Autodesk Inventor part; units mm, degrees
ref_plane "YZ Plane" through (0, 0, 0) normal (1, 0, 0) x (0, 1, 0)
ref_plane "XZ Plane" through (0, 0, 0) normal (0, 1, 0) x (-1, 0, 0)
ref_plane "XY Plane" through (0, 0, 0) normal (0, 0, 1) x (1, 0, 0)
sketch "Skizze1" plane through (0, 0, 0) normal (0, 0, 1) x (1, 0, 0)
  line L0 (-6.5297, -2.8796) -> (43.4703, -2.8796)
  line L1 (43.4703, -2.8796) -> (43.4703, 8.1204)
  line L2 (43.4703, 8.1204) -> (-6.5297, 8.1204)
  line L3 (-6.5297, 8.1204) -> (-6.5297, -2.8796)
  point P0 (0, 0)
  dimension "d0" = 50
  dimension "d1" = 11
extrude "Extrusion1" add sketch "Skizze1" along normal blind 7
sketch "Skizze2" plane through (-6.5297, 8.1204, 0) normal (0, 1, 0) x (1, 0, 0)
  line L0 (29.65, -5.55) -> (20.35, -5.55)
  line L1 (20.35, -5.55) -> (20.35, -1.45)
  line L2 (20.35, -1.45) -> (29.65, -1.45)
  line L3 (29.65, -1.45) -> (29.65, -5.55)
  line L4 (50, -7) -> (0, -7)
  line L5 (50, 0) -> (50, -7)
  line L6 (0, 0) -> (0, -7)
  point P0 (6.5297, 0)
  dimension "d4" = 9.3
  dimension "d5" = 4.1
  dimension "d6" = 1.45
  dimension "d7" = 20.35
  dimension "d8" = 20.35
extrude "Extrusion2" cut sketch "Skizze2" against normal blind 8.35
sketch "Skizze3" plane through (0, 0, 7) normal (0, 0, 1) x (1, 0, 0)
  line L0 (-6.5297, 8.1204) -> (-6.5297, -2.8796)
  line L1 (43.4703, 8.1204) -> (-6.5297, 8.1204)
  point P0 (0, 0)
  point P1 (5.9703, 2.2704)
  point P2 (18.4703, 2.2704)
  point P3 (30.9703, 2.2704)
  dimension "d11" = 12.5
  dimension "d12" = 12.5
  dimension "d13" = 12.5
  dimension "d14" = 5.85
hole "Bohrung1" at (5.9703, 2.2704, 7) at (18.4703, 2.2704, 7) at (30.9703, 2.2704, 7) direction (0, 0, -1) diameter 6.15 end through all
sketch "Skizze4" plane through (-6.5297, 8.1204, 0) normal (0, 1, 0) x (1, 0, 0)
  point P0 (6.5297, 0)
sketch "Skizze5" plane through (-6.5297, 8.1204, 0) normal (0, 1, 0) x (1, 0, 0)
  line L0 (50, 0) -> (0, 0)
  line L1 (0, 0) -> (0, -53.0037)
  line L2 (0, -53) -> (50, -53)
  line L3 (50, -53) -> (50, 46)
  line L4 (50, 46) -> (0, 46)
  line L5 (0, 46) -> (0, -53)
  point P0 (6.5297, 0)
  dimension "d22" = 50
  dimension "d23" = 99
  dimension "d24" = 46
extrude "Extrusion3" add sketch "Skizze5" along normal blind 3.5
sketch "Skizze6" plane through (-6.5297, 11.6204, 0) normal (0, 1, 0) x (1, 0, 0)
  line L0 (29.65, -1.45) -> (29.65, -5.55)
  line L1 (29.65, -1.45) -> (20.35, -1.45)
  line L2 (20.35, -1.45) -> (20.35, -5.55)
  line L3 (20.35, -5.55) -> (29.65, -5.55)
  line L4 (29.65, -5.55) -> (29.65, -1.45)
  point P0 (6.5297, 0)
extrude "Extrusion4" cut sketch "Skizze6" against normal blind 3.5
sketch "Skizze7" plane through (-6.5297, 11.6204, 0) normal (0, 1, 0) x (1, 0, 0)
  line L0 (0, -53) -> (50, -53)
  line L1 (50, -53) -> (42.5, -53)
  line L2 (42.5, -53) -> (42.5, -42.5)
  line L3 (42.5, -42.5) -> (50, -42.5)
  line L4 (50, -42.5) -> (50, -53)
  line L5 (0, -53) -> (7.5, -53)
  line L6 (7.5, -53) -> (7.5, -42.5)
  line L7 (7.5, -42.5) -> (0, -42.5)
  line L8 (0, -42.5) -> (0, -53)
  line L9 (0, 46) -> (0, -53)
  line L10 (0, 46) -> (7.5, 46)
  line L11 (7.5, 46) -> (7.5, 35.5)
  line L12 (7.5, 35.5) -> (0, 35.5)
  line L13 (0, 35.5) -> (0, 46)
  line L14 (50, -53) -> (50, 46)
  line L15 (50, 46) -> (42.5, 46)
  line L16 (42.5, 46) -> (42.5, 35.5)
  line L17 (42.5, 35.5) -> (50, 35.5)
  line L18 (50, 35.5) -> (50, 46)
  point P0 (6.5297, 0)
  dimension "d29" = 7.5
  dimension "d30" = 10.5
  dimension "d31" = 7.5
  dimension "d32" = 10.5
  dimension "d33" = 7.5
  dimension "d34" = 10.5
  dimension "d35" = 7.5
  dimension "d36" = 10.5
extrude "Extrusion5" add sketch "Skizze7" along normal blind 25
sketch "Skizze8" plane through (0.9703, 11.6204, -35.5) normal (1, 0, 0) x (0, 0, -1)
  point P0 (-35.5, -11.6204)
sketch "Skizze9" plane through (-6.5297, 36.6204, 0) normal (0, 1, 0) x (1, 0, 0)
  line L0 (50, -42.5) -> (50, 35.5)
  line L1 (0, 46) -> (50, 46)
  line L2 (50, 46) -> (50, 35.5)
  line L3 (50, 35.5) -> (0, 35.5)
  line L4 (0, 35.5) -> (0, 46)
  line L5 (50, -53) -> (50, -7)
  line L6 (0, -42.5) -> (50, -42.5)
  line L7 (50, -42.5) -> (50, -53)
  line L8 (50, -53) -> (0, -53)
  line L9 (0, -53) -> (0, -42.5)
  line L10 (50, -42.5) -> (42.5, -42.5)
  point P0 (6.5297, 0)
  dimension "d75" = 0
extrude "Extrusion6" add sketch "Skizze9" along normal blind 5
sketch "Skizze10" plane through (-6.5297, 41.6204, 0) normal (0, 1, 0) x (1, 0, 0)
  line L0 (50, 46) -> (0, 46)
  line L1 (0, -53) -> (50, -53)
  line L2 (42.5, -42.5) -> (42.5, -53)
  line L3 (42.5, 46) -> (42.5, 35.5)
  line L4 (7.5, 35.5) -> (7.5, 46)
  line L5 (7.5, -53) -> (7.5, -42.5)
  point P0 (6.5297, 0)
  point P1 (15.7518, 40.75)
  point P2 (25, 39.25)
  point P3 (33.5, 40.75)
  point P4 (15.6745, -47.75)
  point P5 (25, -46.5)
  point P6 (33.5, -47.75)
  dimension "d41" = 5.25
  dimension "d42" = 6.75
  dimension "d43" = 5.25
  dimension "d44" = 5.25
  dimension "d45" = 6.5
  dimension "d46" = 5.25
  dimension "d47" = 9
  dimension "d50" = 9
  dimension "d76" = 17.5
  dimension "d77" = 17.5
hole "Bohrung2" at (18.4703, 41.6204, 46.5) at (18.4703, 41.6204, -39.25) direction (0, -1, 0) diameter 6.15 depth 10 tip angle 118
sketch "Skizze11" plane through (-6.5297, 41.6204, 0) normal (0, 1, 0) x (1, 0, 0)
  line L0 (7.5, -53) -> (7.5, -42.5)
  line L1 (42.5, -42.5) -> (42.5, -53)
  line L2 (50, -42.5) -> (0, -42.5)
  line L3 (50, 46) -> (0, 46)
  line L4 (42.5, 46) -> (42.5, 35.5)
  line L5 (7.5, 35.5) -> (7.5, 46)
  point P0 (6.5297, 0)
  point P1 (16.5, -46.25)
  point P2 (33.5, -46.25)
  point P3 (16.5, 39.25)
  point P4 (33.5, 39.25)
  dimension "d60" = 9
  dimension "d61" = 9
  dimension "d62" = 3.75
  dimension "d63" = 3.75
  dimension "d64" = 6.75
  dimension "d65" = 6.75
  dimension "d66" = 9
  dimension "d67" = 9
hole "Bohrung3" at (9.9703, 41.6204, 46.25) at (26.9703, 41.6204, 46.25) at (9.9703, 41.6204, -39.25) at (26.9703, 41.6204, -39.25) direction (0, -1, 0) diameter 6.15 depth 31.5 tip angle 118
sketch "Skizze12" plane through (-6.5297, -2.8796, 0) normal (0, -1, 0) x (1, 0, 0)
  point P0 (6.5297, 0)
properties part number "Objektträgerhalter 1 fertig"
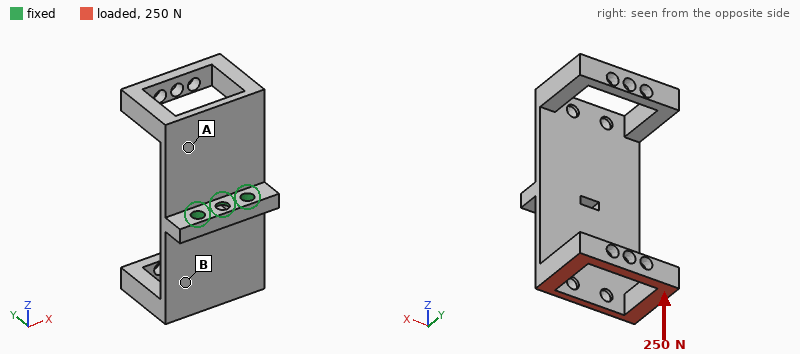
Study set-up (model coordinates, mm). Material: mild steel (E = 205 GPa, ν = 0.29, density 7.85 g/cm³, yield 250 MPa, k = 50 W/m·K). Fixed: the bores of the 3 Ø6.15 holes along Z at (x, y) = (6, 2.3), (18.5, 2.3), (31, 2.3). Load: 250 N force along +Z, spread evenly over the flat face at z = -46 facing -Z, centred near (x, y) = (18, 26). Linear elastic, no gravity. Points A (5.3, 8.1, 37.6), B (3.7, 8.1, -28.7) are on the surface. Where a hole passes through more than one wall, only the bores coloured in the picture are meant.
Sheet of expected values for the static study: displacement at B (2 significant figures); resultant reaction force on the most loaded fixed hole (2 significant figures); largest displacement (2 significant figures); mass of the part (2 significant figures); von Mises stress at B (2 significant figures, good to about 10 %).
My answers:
0.053 mm
150 N
0.20 mm
250 g
35 MPa
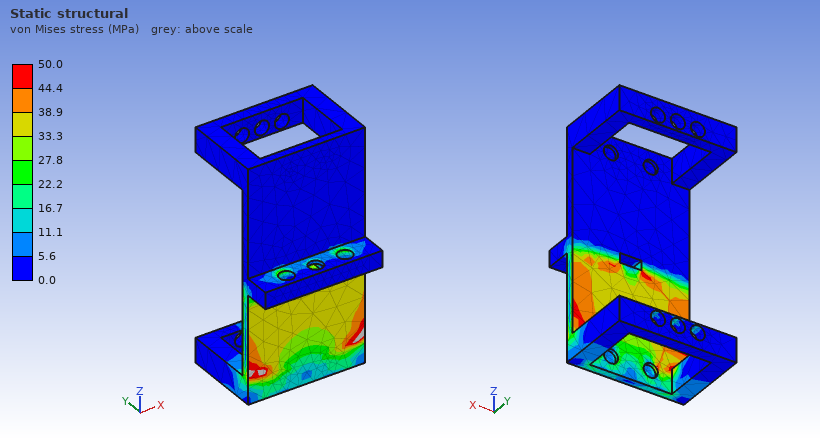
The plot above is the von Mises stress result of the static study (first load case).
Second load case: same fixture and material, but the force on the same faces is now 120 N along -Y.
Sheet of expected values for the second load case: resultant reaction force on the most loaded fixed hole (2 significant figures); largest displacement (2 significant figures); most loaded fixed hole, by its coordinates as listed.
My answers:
92 N
0.17 mm
(18.5, 2.3)
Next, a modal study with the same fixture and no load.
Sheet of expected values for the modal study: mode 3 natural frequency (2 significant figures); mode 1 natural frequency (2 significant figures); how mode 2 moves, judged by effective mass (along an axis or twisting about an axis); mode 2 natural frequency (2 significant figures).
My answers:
1100 Hz
570 Hz
along Y
600 Hz
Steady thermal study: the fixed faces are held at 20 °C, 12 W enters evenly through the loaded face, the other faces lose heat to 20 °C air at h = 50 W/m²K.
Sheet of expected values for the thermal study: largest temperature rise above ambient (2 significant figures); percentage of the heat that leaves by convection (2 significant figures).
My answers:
40 K
70 %
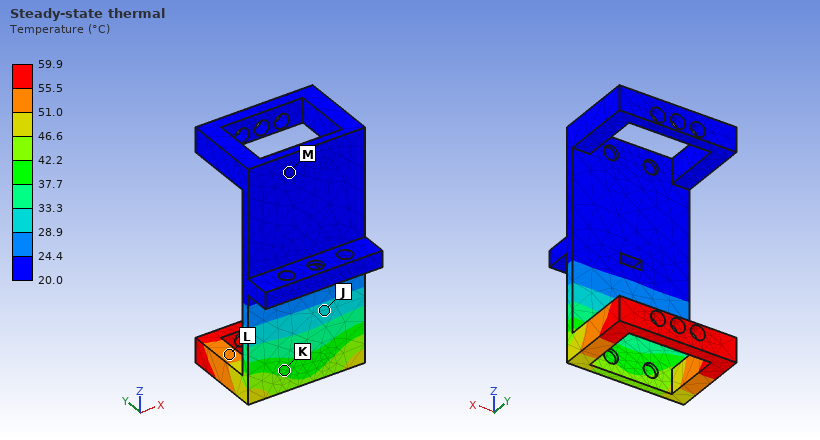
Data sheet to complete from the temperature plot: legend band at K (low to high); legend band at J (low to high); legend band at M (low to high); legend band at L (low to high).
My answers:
37.7 to 42.2 °C
28.9 to 33.3 °C
20.0 to 24.4 °C
51.0 to 55.5 °C
